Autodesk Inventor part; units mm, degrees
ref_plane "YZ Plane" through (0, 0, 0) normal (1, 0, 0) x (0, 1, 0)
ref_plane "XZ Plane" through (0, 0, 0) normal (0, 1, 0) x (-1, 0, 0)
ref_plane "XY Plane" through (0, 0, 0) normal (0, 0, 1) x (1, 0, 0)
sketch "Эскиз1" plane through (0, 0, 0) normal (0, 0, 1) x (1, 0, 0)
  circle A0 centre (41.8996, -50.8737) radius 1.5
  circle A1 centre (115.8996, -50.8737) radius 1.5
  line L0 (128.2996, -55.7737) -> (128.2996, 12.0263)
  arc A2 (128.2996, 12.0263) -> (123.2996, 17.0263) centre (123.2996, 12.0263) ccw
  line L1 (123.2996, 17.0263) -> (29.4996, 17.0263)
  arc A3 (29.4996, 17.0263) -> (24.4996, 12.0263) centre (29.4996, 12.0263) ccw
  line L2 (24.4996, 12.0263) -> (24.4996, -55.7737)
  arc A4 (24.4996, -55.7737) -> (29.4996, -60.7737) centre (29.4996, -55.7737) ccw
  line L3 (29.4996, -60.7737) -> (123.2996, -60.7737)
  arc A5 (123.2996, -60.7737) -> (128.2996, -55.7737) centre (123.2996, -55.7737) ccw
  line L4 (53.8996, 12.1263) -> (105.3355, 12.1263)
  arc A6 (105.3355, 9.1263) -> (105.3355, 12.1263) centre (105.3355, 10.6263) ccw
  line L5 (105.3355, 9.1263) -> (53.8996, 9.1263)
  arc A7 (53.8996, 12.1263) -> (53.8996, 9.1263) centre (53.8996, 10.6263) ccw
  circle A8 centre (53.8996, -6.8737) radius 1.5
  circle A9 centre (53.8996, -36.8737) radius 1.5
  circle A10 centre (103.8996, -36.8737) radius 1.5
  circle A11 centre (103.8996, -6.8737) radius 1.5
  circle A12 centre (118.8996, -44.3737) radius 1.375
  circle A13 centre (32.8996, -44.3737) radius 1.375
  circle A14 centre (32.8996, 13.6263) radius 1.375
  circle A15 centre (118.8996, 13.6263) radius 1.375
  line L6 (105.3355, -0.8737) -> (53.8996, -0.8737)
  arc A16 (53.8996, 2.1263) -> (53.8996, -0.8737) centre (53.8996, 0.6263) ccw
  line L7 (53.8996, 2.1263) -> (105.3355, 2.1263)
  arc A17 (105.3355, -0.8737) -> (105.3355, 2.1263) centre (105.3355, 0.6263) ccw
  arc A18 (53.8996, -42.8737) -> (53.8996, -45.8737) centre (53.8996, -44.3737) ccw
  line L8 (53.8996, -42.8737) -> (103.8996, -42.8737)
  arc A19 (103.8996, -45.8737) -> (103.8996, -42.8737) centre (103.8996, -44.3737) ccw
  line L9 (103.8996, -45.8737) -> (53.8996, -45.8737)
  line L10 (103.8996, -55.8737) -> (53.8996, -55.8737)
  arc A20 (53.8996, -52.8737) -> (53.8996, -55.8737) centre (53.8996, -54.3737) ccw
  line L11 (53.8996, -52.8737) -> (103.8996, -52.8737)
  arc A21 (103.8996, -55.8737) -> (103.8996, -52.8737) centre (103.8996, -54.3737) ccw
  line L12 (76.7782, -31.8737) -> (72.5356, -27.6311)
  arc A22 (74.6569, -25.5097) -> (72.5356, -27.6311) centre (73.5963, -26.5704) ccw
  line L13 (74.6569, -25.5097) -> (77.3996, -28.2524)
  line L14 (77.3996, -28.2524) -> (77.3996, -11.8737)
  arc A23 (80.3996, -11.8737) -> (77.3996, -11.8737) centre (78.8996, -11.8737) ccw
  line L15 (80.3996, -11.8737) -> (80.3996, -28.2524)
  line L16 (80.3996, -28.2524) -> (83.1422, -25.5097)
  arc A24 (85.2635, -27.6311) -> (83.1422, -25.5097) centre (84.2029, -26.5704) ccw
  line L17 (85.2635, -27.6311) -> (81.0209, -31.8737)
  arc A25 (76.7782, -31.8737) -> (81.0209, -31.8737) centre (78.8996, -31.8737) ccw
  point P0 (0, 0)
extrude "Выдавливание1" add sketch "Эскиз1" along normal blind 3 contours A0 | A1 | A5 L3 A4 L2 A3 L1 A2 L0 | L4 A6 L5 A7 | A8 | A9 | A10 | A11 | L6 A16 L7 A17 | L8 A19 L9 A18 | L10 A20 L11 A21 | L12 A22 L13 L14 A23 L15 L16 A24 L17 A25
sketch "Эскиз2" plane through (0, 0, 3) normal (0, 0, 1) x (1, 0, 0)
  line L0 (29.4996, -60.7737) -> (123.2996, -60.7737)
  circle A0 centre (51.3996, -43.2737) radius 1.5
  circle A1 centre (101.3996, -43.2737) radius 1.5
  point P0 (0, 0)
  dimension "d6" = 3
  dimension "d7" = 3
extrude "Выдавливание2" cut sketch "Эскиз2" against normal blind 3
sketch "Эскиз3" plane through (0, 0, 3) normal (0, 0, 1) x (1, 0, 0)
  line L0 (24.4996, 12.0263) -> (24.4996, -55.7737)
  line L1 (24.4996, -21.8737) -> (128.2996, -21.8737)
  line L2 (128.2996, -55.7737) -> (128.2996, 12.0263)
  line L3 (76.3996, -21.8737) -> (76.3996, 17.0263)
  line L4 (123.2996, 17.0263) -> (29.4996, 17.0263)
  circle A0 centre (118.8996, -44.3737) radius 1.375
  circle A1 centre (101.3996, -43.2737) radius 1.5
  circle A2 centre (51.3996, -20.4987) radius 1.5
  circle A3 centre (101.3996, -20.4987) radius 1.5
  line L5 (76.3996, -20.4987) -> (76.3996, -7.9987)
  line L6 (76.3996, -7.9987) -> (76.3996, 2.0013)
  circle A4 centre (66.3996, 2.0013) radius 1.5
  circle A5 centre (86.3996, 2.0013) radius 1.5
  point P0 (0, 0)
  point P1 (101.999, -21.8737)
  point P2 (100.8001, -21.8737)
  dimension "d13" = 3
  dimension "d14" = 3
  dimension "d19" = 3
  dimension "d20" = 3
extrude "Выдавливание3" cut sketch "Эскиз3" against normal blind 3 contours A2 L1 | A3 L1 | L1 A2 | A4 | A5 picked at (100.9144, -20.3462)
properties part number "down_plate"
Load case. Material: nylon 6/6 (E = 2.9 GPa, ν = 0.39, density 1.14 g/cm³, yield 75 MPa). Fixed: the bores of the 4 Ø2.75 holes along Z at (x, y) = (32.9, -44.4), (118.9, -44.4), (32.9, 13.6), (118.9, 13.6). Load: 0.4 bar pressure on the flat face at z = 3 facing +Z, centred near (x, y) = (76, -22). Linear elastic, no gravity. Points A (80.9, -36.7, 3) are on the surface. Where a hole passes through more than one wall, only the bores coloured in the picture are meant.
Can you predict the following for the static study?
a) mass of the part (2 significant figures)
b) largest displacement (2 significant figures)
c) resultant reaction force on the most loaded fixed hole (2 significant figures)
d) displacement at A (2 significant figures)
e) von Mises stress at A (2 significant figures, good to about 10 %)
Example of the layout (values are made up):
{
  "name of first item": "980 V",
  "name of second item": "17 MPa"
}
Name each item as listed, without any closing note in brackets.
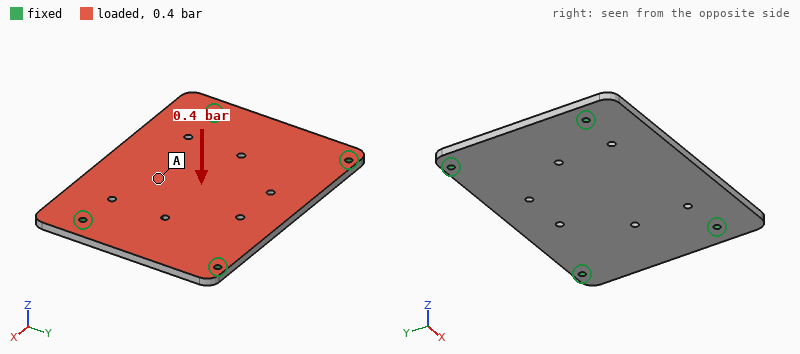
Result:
{
  "mass of the part": "27 g",
  "largest displacement": "1.4 mm",
  "resultant reaction force on the most loaded fixed hole": "96 N",
  "displacement at A": "1.2 mm",
  "von Mises stress at A": "8.9 MPa"
}
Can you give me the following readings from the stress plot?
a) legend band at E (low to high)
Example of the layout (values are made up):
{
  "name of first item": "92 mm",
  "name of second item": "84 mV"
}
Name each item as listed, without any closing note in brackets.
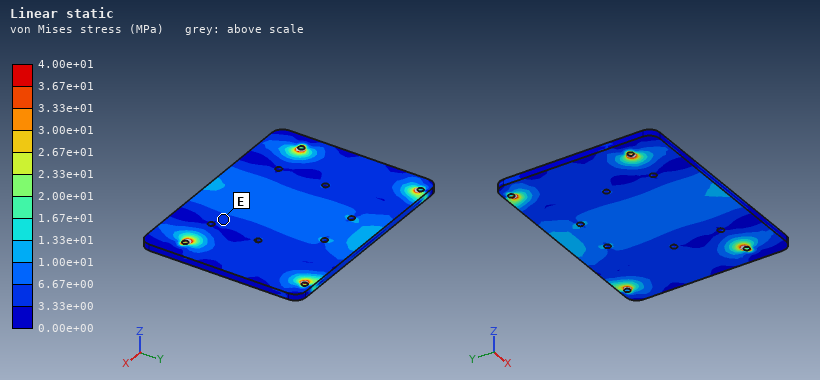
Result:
{
  "legend band at E": "3.33e+00 to 6.67e+00 MPa"
}
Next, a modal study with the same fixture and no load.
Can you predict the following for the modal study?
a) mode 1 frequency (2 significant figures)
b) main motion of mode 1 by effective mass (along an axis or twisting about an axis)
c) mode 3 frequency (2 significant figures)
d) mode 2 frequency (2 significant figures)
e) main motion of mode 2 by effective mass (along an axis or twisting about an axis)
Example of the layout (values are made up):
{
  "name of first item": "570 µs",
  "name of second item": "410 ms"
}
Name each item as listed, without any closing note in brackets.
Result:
{
  "mode 1 frequency": "540 Hz",
  "main motion of mode 1 by effective mass": "along Z",
  "mode 3 frequency": "1200 Hz",
  "mode 2 frequency": "740 Hz",
  "main motion of mode 2 by effective mass": "twisting about X"
}
